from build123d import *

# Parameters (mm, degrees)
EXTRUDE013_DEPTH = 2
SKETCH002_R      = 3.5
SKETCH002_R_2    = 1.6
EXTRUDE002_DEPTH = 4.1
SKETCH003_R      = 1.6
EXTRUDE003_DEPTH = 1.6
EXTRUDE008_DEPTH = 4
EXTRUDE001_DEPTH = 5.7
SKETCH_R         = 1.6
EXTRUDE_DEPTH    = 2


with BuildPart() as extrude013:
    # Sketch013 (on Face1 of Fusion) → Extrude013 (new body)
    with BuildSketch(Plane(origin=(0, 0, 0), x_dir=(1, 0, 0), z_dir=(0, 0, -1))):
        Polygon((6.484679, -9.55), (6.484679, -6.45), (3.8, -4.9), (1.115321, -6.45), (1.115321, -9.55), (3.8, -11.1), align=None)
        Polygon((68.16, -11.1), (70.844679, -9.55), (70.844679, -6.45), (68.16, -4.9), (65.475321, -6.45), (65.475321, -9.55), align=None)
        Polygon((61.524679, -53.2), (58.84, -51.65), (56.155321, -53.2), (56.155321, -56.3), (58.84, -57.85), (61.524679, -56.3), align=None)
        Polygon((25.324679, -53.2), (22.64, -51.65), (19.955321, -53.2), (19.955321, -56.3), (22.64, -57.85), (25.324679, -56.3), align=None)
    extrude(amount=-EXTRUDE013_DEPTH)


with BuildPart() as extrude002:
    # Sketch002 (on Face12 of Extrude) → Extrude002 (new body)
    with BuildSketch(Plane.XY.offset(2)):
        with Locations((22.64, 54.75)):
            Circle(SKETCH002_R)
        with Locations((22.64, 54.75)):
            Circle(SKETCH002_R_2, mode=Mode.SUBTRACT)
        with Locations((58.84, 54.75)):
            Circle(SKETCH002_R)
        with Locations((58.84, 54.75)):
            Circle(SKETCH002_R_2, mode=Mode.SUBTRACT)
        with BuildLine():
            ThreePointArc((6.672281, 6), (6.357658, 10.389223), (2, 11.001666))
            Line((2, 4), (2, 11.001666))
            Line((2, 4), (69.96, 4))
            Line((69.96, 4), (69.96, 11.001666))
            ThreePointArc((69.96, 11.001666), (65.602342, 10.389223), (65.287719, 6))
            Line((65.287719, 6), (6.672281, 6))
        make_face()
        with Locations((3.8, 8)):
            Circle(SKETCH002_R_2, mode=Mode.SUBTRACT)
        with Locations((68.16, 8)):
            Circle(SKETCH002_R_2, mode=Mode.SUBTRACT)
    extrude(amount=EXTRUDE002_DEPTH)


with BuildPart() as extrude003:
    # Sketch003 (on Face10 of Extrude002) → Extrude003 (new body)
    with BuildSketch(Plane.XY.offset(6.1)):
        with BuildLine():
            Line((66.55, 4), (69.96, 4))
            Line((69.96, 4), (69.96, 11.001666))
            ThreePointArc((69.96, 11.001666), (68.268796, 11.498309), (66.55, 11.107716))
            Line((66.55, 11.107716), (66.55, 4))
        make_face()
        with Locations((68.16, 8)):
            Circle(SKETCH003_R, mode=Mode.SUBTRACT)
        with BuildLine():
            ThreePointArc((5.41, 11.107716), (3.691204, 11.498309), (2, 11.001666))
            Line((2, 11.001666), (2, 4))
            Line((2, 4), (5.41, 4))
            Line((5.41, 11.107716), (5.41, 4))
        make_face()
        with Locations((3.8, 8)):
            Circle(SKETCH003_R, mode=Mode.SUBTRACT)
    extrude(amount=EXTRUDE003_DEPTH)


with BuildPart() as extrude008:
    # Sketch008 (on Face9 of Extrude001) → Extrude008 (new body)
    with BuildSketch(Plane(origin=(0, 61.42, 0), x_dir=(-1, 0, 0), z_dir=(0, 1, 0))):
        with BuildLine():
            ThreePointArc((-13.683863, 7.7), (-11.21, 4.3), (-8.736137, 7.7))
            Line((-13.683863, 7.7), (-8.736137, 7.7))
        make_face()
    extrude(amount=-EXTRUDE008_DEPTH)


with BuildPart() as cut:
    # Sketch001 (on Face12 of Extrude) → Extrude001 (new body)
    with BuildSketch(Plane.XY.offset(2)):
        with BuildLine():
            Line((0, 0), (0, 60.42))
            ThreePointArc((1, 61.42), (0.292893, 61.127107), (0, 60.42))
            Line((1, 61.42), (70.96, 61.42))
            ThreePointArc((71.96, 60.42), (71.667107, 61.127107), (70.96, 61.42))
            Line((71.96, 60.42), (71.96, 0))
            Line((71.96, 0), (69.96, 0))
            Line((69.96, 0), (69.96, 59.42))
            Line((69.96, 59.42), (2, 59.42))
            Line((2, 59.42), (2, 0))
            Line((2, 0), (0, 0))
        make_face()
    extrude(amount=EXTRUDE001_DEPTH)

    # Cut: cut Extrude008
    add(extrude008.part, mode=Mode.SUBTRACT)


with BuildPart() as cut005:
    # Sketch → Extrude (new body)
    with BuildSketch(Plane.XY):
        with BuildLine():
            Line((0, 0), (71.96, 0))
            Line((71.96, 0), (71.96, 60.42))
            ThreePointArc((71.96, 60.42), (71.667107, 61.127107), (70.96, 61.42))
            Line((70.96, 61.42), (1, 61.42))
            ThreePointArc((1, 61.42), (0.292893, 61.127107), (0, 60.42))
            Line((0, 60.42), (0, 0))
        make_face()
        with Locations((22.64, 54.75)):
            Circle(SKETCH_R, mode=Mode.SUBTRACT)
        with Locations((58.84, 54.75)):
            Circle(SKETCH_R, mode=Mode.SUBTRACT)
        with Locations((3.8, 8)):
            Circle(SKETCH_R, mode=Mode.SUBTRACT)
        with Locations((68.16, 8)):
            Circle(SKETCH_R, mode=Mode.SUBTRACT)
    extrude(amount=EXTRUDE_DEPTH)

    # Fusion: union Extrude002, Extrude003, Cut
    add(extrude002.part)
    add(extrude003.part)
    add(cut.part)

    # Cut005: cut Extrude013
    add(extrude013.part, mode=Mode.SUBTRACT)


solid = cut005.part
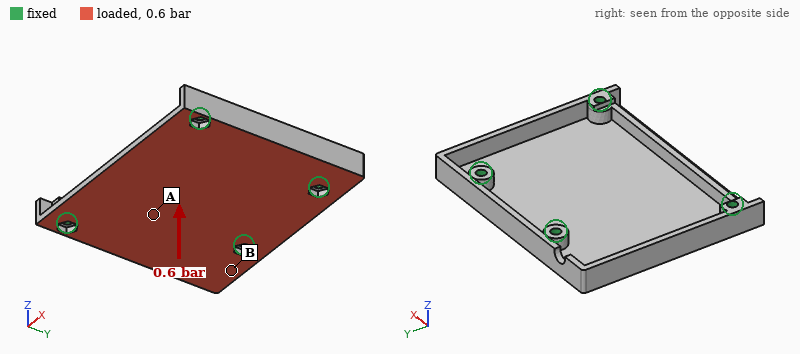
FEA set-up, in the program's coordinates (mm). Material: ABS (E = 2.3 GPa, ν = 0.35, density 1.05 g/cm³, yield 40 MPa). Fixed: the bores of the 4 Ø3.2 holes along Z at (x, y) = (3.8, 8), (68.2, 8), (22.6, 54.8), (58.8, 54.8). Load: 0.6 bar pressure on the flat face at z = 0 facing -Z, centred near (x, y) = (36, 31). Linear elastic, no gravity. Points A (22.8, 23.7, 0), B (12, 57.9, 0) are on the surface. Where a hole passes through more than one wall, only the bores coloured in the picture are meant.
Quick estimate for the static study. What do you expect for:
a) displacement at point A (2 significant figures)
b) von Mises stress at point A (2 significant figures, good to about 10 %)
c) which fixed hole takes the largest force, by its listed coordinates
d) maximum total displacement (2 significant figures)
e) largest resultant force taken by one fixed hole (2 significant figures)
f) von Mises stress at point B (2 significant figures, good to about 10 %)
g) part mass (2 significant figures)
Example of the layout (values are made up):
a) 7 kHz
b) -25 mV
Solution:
a) 0.76 mm
b) 8.5 MPa
c) (3.8, 8)
d) 0.95 mm
e) 120 N
f) 2.4 MPa
g) 12 g
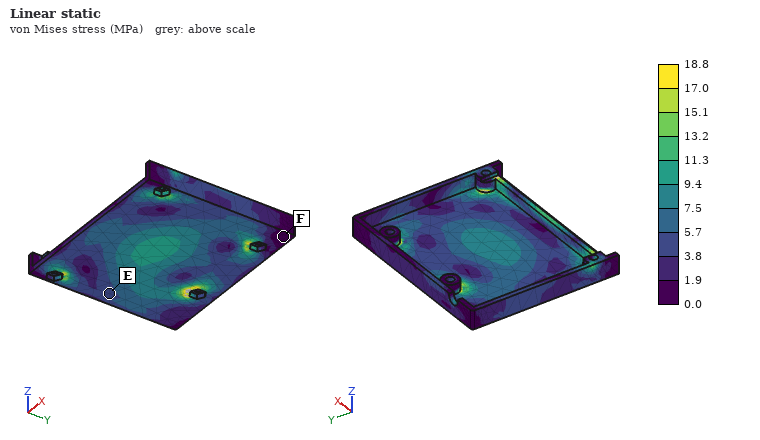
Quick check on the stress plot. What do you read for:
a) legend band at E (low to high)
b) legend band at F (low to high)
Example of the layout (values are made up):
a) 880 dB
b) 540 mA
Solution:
a) 3.8 to 5.7 MPa
b) 0.0 to 1.9 MPa
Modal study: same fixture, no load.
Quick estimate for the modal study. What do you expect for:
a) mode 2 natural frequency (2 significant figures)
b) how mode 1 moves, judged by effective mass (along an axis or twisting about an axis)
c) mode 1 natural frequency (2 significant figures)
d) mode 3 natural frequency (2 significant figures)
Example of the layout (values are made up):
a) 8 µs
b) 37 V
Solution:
a) 1400 Hz
b) along Z
c) 1100 Hz
d) 1800 Hz
